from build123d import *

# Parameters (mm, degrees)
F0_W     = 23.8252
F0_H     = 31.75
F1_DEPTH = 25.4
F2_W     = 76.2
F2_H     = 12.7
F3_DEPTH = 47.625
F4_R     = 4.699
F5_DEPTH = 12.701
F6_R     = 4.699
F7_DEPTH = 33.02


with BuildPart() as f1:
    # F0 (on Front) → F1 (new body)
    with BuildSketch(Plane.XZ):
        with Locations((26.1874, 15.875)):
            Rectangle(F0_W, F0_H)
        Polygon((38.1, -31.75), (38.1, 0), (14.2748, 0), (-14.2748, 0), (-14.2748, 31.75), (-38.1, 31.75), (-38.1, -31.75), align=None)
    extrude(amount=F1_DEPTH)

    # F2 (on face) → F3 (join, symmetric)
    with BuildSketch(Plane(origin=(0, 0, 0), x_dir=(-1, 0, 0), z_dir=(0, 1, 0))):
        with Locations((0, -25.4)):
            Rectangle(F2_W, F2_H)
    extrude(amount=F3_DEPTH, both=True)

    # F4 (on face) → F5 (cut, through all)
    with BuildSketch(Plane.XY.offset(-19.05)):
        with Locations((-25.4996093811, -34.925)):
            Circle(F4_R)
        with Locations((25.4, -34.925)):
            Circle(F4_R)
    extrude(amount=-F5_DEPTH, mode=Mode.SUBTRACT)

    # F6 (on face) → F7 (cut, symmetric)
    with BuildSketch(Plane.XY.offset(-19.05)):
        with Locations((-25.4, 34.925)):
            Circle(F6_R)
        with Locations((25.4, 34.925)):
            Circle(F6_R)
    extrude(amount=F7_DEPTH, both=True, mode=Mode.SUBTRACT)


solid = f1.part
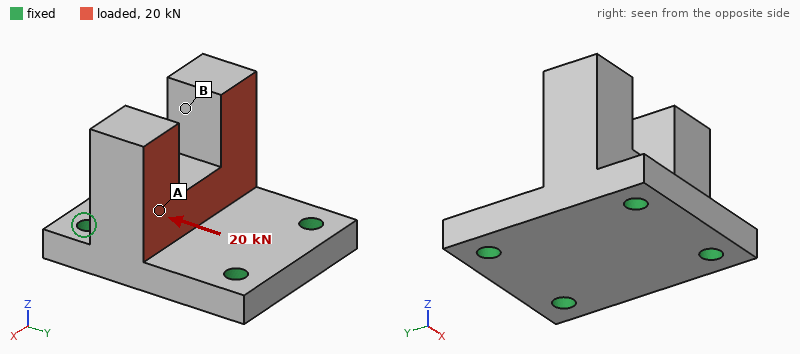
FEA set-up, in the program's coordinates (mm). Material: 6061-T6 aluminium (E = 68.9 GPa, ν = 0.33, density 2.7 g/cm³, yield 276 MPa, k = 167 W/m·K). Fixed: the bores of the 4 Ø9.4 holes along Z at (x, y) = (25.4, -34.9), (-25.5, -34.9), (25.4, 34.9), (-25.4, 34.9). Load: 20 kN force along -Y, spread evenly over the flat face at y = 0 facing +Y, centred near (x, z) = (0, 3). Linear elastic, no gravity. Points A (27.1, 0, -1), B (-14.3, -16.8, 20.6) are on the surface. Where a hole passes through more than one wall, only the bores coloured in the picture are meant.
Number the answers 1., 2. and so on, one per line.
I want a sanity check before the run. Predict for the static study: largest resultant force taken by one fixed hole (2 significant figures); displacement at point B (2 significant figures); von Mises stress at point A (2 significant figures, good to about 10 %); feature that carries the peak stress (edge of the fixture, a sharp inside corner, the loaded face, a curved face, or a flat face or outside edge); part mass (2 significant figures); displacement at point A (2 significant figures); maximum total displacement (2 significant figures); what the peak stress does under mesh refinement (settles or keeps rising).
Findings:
1. 8.1 kN
2. 0.14 mm
3. 33 MPa
4. edge of the fixture
5. 440 g
6. 0.087 mm
7. 0.18 mm
8. keeps rising
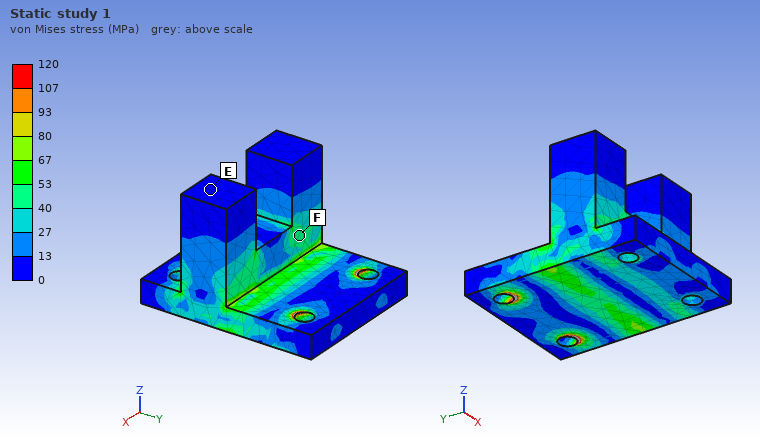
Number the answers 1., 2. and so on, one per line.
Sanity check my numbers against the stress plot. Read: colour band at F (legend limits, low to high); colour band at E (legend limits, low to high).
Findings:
1. 40 to 53 MPa
2. 0 to 13 MPa
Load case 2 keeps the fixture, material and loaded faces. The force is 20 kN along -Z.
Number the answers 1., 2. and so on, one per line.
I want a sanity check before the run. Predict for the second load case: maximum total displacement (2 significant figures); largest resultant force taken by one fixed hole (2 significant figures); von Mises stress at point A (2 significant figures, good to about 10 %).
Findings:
1. 0.15 mm
2. 5.1 kN
3. 34 MPa
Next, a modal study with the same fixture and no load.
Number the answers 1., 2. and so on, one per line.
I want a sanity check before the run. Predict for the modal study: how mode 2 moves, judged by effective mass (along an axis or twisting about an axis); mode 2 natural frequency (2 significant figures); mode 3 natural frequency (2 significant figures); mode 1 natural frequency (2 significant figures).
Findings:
1. along X
2. 5000 Hz
3. 6300 Hz
4. 4400 Hz
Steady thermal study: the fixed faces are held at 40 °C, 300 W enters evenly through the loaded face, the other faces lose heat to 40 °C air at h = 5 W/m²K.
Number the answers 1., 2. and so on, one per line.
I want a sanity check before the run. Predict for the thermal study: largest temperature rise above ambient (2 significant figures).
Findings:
1. 57 K
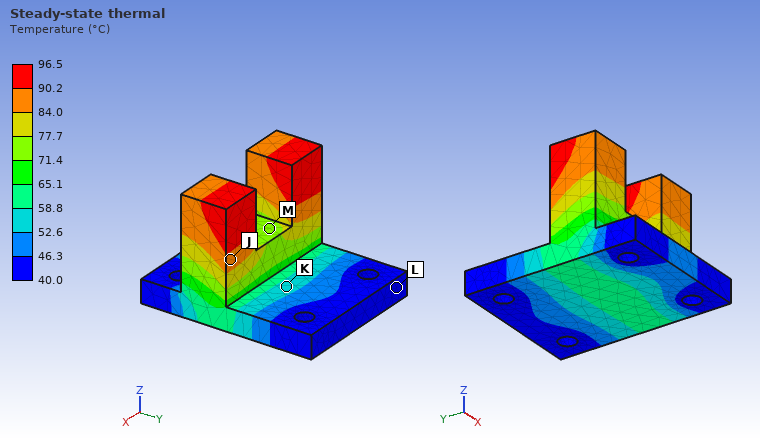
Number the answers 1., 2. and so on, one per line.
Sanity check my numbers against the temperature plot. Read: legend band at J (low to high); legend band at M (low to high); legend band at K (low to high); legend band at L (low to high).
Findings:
1. 84.0 to 90.2 °C
2. 71.4 to 77.7 °C
3. 52.6 to 58.8 °C
4. 40.0 to 46.3 °C
